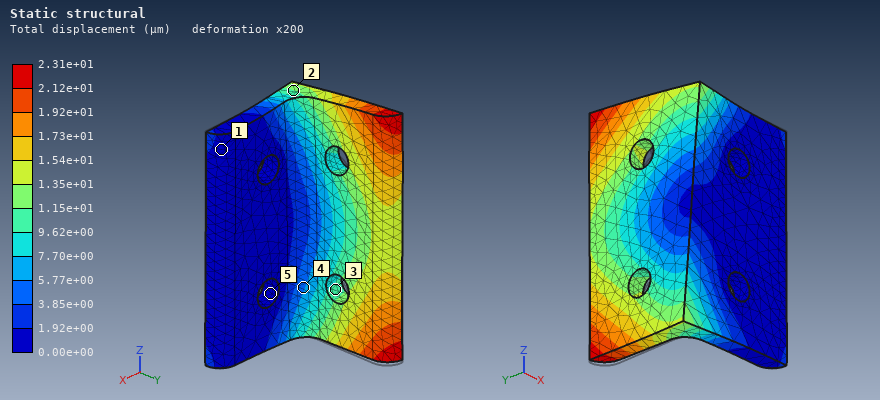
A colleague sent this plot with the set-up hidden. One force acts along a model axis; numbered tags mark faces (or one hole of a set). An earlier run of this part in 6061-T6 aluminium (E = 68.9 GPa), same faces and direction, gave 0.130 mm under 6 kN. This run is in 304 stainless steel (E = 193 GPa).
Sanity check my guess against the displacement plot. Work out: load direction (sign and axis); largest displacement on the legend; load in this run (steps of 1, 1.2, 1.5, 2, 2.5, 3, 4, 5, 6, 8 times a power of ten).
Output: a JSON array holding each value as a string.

["+Z", "2.31e+01 µm", "3 kN"]
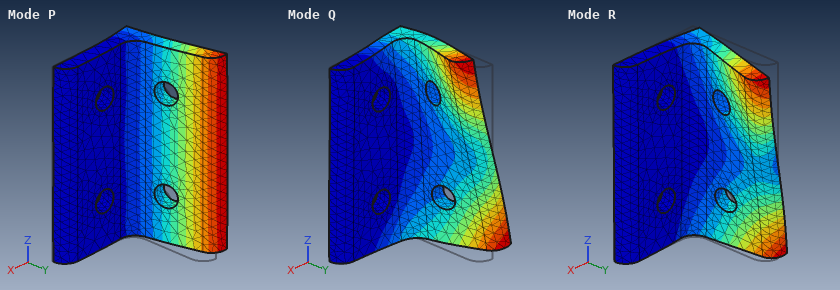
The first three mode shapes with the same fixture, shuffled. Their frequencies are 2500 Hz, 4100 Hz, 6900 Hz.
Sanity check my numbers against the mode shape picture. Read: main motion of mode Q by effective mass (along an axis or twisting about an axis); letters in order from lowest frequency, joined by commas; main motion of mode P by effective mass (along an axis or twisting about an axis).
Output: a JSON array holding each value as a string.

["along Z", "P, R, Q", "along X"]
